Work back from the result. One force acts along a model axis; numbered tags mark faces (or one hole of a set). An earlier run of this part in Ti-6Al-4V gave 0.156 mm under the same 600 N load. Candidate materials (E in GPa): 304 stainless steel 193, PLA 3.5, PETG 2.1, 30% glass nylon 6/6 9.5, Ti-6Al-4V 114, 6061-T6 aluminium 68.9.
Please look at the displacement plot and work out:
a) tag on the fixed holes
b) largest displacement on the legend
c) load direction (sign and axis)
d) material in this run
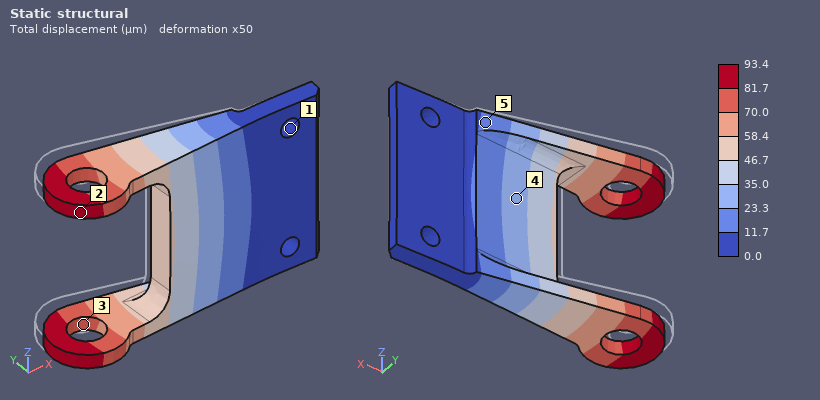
1
93.4 µm
-Y
304 stainless steel
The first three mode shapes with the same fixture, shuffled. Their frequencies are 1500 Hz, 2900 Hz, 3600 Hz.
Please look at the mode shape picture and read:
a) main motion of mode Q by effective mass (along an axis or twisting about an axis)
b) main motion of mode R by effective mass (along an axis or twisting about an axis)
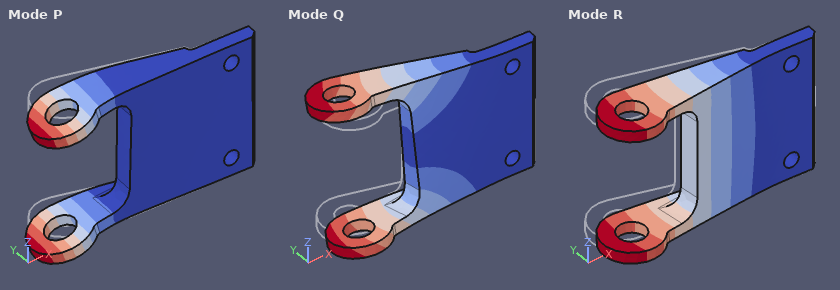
twisting about X
along Y
